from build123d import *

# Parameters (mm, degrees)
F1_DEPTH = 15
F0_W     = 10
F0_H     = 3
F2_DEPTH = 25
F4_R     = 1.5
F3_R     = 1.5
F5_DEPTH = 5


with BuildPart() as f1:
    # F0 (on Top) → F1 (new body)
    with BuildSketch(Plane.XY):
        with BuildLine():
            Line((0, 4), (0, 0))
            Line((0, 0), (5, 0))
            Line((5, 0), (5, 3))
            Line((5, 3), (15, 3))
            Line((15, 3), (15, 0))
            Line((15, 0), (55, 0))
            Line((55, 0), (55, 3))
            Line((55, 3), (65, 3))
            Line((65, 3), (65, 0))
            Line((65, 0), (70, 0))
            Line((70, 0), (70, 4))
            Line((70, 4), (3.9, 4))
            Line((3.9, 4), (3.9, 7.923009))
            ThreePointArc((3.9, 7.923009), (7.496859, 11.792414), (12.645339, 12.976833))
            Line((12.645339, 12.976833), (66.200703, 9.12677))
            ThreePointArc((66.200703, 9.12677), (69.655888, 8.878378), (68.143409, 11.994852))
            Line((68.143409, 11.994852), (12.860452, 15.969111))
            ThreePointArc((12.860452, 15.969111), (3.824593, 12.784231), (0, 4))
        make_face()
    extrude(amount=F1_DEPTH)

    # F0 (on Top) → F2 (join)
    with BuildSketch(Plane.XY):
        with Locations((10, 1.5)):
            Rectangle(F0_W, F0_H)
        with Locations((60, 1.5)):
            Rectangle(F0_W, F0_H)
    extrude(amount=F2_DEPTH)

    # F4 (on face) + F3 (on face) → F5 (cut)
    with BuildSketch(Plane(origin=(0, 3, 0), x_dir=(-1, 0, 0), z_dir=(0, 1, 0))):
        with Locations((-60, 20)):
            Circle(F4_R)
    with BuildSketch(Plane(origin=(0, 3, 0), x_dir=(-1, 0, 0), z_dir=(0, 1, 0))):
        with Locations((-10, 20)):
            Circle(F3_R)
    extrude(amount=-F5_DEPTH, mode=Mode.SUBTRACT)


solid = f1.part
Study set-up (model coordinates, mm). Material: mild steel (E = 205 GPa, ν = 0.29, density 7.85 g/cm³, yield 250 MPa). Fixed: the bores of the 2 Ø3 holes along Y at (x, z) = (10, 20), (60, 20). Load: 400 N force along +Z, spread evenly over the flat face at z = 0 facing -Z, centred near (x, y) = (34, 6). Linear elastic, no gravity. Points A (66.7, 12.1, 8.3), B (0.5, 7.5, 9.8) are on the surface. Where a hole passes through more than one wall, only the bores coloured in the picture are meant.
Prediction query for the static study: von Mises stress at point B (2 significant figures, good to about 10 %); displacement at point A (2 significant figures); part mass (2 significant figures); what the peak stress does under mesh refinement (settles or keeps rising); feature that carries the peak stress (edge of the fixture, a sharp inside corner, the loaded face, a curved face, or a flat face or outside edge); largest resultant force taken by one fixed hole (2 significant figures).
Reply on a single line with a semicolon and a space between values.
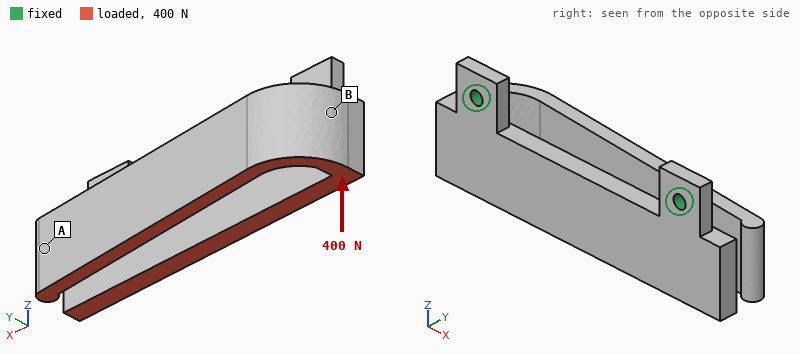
120 MPa; 0.28 mm; 64 g; keeps rising; edge of the fixture; 270 N
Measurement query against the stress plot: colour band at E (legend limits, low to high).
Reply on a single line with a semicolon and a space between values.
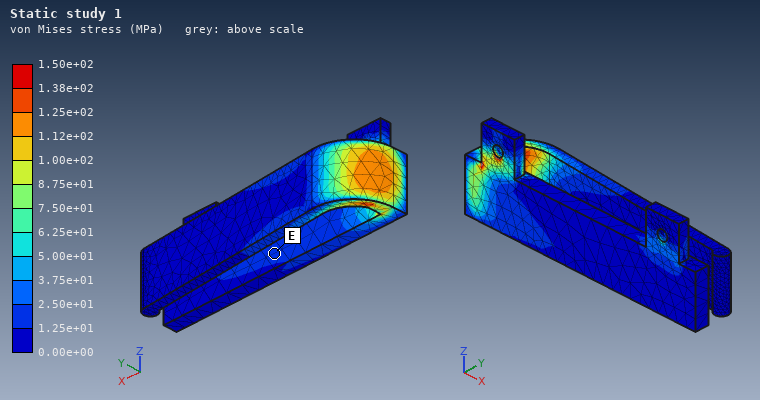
1.25e+01 to 2.50e+01 MPa
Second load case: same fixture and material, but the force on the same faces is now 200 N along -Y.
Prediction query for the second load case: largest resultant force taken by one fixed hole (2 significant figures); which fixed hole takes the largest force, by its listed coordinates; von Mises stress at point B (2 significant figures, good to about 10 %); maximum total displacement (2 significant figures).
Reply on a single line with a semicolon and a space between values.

120 N; (10, 20); 74 MPa; 0.77 mm
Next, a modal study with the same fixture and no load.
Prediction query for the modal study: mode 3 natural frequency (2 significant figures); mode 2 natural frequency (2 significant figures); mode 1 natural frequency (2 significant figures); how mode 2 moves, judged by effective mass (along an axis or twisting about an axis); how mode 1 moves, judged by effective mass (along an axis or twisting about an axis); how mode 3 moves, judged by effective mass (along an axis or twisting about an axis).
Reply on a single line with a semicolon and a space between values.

2200 Hz; 920 Hz; 420 Hz; along Z; along Y; along Y
